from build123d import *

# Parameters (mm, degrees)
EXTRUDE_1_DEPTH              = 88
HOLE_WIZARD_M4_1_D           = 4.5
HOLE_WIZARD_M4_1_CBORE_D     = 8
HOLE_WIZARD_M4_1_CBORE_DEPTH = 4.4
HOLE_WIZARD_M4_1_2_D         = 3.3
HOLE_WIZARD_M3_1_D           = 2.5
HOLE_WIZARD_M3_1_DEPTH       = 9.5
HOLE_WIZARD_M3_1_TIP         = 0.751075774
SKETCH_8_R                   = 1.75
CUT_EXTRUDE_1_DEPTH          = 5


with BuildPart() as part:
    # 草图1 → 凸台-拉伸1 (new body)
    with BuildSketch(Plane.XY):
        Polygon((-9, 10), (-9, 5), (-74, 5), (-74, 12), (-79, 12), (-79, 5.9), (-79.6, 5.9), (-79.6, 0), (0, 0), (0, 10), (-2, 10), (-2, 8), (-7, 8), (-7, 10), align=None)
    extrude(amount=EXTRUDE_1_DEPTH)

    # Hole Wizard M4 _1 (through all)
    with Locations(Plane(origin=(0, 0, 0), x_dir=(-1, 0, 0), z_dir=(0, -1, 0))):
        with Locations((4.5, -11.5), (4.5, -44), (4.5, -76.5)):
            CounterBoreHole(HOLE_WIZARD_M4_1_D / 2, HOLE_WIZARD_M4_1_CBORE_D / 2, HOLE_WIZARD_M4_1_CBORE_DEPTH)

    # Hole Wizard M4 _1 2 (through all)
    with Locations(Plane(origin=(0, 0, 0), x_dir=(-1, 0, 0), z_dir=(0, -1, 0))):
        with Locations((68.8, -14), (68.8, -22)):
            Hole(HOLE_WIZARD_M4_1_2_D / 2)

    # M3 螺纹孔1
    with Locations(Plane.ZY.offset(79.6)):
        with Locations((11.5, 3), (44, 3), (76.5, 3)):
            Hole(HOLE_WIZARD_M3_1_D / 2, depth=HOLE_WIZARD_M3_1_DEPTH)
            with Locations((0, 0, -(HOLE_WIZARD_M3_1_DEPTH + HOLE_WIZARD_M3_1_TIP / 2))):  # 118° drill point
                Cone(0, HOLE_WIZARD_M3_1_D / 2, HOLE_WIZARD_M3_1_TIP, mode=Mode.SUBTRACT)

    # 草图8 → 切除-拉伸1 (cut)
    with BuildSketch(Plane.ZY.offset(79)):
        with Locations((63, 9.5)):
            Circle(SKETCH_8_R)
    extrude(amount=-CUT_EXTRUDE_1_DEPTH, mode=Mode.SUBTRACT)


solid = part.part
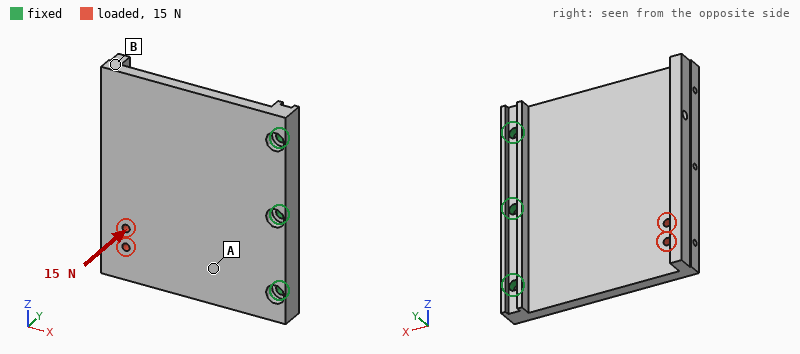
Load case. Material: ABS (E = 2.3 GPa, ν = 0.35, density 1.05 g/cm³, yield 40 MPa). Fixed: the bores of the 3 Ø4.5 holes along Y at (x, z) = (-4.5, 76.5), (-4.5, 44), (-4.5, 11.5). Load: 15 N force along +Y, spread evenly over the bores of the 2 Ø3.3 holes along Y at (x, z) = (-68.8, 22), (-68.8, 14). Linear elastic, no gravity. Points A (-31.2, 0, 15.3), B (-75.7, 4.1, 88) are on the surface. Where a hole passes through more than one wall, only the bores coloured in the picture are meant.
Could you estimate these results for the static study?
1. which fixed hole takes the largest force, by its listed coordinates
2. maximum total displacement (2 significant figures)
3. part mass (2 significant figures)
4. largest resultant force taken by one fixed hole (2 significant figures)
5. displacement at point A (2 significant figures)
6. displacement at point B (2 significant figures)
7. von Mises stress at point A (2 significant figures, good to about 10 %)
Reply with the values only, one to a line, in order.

(-4.5, 44)
1.2 mm
42 g
12 N
0.25 mm
0.63 mm
1.7 MPa
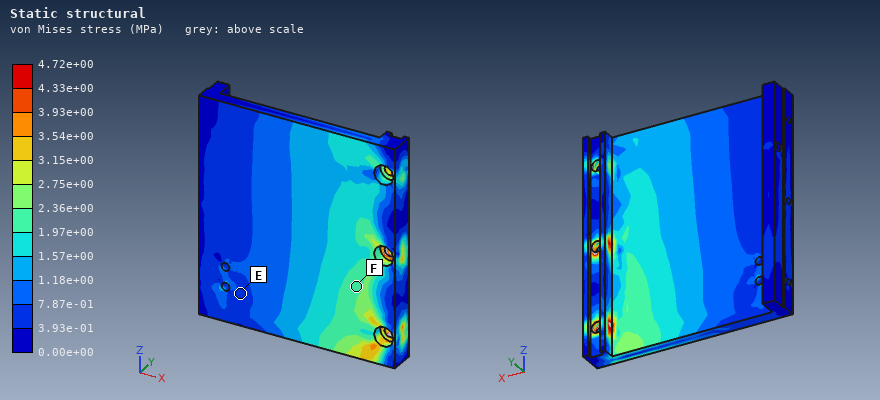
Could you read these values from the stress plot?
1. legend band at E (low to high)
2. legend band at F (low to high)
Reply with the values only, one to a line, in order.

3.93e-01 to 7.87e-01 MPa
1.97e+00 to 2.36e+00 MPa
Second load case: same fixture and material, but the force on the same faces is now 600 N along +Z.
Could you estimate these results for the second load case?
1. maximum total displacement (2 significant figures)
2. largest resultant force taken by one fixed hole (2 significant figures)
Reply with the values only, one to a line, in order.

0.74 mm
600 N
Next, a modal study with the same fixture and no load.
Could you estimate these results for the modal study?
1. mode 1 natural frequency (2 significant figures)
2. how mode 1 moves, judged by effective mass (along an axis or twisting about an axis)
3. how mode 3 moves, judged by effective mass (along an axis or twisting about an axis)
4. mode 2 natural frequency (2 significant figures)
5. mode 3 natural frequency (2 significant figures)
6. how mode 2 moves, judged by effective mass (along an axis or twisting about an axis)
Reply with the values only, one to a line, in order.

170 Hz
along Y
along Y
400 Hz
1100 Hz
twisting about X
